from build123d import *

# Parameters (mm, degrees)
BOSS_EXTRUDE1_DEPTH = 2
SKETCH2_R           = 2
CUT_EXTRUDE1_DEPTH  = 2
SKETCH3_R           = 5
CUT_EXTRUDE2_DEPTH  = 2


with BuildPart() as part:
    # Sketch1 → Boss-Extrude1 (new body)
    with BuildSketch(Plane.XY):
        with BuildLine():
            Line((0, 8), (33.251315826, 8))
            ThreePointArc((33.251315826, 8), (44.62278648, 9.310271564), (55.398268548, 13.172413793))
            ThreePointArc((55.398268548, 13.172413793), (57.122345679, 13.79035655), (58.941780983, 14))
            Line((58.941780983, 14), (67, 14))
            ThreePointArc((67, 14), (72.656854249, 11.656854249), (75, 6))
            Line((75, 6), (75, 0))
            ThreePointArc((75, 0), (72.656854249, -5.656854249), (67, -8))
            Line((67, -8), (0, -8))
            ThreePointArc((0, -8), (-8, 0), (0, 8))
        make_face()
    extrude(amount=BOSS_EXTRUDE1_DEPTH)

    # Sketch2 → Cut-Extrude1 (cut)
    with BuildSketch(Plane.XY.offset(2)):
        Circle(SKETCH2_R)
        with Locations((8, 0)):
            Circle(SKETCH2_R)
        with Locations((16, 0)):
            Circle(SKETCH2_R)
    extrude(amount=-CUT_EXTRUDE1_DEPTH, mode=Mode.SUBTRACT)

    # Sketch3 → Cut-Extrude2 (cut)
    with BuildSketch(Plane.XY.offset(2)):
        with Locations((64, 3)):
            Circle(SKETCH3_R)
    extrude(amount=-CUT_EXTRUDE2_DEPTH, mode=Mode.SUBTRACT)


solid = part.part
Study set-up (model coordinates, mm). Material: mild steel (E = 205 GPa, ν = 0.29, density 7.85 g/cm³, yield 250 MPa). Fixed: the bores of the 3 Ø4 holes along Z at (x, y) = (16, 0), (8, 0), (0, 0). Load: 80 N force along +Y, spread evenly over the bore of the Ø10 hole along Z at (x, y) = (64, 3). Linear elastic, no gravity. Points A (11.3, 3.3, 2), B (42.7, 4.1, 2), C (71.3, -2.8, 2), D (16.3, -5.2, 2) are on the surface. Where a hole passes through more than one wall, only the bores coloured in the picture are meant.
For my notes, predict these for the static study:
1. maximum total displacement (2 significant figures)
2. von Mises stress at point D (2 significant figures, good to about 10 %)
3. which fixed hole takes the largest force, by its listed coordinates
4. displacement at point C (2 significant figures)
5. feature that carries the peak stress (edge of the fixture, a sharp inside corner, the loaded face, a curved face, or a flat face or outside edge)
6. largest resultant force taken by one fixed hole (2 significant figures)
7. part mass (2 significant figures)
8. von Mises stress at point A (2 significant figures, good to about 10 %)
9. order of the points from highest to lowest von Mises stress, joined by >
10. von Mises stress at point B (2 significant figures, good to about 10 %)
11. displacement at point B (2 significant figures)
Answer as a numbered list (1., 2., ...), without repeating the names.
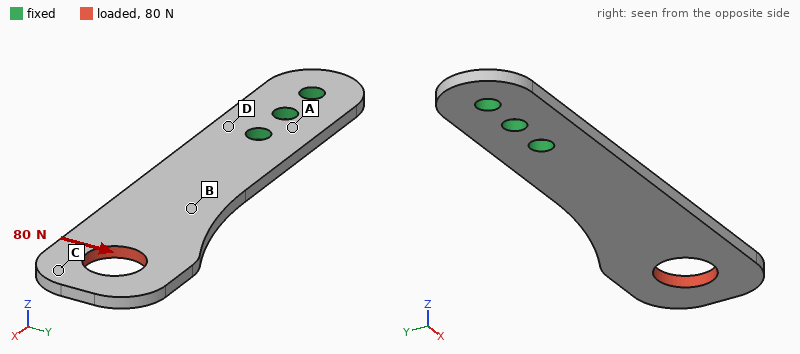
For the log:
1. 38 µm
2. 26 MPa
3. (16, 0)
4. 35 µm
5. edge of the fixture
6. 280 N
7. 21 g
8. 17 MPa
9. D > A > B > C
10. 9.3 MPa
11. 13 µm
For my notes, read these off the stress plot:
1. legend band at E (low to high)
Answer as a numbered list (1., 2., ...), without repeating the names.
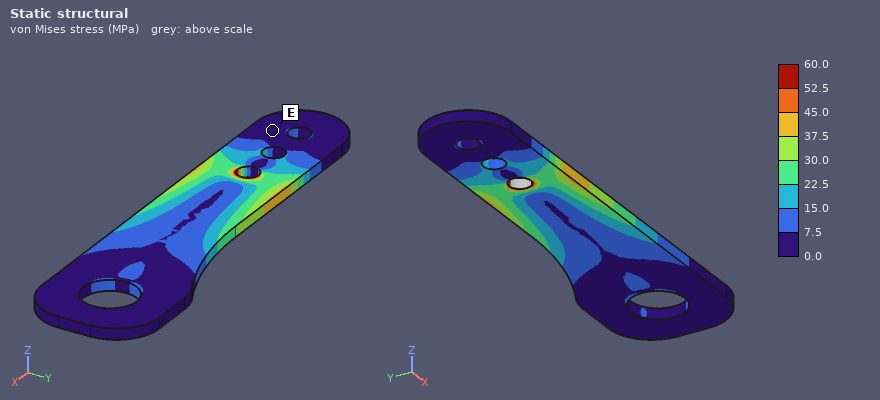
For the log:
1. 0.0 to 7.5 MPa
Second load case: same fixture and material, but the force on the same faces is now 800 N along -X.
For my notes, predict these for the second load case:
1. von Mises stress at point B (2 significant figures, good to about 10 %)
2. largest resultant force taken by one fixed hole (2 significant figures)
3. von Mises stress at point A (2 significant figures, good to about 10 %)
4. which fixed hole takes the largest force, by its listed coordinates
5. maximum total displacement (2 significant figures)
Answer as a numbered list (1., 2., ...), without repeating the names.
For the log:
1. 31 MPa
2. 640 N
3. 20 MPa
4. (16, 0)
5. 31 µm
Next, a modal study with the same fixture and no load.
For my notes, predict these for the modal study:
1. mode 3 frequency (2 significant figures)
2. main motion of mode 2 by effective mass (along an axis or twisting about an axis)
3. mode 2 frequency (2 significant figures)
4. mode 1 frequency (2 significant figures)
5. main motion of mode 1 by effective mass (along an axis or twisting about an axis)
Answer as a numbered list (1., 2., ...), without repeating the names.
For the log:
1. 3000 Hz
2. twisting about X
3. 2500 Hz
4. 480 Hz
5. along Z
